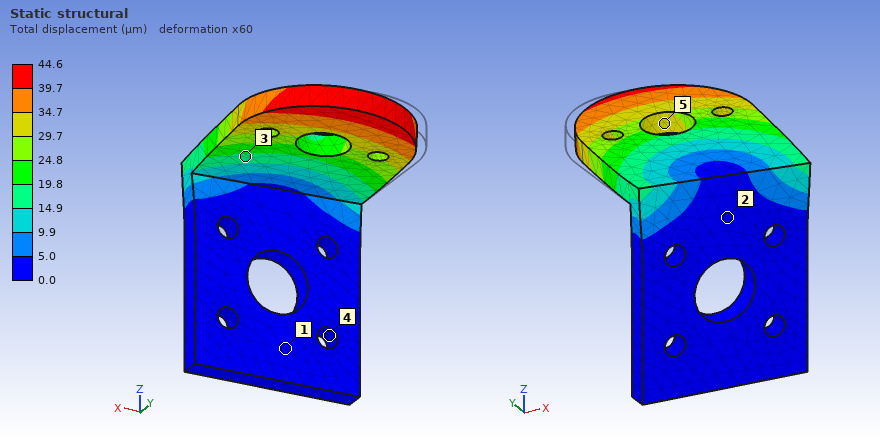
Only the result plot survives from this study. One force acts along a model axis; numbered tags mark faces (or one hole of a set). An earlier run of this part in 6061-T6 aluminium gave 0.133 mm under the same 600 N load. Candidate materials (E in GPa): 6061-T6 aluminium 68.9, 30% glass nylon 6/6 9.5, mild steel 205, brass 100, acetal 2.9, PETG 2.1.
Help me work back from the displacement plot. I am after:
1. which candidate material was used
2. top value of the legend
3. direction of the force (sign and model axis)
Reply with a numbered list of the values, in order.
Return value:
1. mild steel
2. 44.6 µm
3. +X
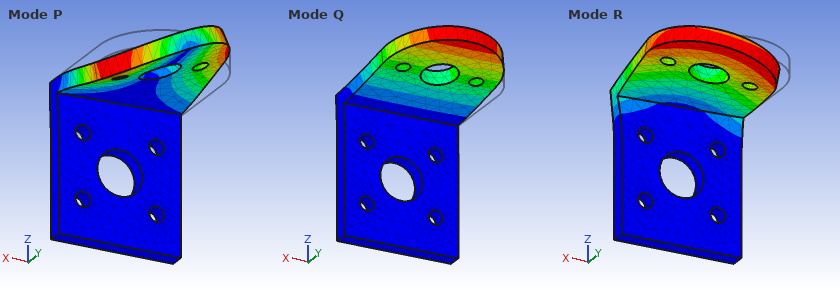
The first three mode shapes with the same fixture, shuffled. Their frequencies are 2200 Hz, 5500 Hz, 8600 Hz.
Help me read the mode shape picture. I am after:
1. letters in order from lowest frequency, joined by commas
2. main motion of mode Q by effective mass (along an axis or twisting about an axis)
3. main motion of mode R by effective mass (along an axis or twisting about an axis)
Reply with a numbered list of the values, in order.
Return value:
1. Q, R, P
2. along Z
3. along X
